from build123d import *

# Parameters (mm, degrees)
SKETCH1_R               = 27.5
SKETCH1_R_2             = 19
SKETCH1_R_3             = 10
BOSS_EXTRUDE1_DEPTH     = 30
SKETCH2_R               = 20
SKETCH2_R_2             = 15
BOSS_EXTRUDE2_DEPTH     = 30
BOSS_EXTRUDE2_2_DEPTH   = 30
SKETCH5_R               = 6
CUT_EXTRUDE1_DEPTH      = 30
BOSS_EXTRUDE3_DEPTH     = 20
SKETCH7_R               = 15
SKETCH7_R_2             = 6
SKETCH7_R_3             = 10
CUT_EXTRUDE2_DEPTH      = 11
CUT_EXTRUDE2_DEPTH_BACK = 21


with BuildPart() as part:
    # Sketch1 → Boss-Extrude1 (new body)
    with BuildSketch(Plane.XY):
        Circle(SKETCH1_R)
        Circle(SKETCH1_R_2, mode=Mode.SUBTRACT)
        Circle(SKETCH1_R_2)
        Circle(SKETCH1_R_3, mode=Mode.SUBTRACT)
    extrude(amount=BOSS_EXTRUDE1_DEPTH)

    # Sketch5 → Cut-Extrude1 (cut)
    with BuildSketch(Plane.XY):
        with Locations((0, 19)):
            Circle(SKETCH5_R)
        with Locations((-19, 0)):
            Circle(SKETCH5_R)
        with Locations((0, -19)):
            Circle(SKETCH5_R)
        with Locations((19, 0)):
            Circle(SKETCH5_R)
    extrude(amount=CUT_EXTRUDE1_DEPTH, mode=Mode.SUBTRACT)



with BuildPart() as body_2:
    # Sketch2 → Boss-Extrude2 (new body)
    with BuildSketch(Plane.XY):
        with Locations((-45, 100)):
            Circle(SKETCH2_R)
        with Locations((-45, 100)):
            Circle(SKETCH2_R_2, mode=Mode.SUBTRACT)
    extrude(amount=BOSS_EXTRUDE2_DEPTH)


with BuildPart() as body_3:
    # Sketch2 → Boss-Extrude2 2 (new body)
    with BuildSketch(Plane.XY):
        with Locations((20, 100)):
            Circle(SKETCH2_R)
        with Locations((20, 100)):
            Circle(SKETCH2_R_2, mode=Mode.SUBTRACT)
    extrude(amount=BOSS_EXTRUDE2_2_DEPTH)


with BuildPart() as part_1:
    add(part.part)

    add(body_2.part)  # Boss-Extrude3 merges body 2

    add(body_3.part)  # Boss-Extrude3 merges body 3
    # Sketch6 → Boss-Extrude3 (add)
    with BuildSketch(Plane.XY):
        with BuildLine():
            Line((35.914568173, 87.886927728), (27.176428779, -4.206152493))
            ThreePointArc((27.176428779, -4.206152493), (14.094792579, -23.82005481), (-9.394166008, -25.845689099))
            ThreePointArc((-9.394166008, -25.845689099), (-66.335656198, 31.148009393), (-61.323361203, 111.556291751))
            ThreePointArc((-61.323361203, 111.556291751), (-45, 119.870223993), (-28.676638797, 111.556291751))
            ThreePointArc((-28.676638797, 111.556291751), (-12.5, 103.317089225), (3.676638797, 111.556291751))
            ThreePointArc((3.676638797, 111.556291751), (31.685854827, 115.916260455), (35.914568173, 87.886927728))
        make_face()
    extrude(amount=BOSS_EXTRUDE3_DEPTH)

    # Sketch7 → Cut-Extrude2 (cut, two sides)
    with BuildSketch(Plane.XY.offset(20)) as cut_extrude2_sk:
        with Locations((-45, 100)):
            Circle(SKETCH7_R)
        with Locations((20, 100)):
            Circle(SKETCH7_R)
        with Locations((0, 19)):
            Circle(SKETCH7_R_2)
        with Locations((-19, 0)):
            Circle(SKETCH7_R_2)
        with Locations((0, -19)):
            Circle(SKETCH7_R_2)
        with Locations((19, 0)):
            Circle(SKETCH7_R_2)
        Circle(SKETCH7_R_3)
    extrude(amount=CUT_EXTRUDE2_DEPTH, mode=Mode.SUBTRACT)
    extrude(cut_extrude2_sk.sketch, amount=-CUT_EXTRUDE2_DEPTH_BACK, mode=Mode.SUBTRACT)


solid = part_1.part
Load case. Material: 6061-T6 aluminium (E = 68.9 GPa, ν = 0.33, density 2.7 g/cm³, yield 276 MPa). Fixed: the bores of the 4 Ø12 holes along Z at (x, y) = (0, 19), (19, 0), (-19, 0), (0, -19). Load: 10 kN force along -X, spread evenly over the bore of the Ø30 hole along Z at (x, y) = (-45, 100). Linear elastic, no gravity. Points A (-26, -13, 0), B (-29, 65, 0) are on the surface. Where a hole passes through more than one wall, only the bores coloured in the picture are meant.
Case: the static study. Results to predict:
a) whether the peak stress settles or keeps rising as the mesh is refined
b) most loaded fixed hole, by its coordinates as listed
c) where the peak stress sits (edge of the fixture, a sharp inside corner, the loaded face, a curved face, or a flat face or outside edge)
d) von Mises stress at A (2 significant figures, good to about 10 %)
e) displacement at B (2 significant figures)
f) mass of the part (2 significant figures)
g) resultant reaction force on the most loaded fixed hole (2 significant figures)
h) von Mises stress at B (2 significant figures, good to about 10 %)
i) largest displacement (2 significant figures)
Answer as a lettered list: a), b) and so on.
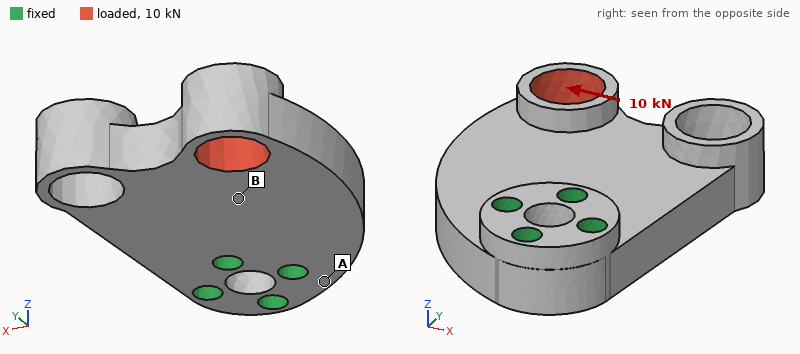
a) keeps rising
b) (0, 19)
c) a sharp inside corner
d) 23 MPa
e) 0.043 mm
f) 640 g
g) 18 kN
h) 6.8 MPa
i) 0.16 mm
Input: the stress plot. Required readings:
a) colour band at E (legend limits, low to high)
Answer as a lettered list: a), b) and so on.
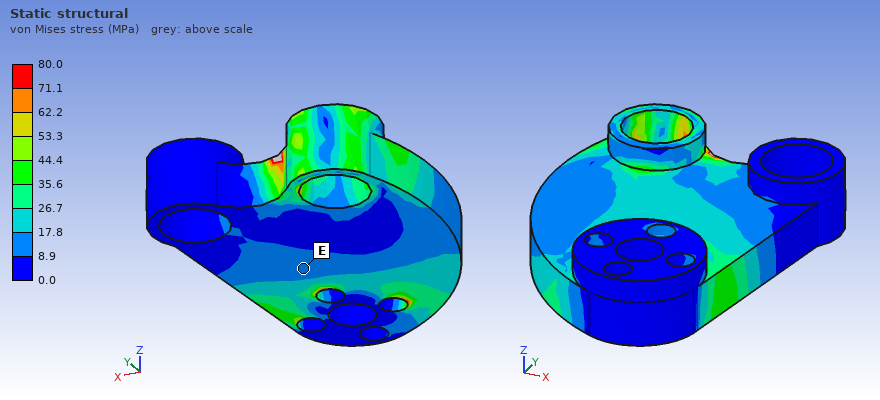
a) 8.9 to 17.8 MPa
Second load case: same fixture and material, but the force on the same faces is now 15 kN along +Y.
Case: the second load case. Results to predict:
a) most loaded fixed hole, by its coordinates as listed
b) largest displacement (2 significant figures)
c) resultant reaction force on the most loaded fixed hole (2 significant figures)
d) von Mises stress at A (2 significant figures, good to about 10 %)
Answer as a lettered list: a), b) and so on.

a) (-19, 0)
b) 0.17 mm
c) 16 kN
d) 21 MPa
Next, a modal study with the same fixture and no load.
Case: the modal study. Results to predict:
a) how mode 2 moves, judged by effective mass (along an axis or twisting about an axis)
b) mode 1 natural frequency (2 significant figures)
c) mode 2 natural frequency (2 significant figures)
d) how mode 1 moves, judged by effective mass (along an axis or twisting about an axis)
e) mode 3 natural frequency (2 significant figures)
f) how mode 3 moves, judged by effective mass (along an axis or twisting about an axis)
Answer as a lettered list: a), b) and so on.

a) twisting about Y
b) 1700 Hz
c) 2800 Hz
d) along Z
e) 3600 Hz
f) along X
